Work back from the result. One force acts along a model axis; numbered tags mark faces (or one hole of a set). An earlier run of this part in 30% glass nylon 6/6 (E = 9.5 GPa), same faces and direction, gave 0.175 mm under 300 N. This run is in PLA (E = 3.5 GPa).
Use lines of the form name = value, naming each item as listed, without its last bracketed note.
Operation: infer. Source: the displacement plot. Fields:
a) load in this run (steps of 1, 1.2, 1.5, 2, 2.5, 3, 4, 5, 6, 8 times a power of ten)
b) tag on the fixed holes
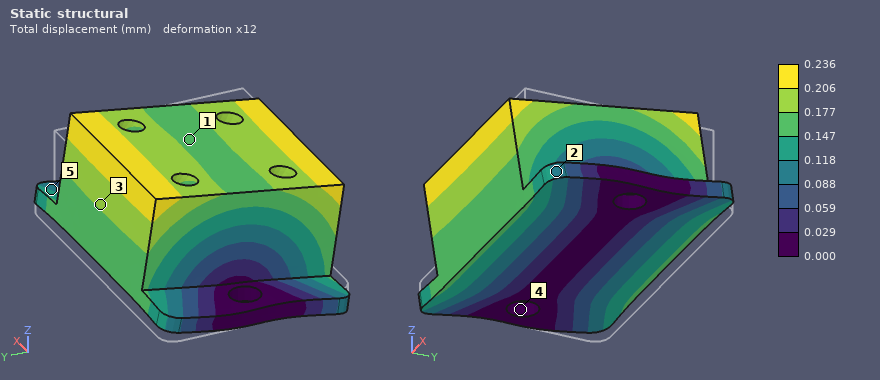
load in this run = 150 N
tag on the fixed holes = 4
